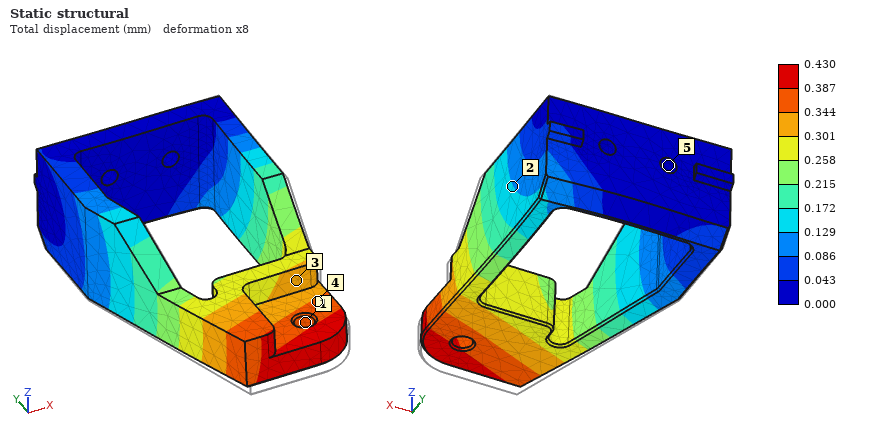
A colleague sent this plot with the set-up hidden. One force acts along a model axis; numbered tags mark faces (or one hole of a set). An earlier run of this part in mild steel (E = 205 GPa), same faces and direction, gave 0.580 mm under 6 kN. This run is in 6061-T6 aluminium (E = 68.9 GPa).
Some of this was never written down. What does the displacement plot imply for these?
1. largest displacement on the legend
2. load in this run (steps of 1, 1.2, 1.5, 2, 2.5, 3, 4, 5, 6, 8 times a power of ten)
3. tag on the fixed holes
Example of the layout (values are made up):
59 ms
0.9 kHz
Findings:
0.430 mm
1.5 kN
5
